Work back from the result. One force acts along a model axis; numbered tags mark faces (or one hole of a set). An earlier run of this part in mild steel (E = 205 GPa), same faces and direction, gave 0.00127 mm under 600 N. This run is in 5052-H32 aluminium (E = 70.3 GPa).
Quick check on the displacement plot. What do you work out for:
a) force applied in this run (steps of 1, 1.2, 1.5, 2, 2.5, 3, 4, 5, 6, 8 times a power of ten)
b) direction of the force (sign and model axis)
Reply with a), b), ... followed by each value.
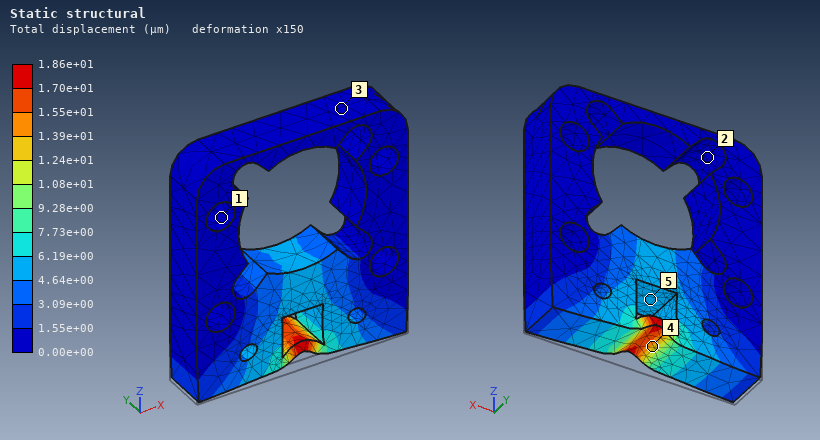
a) 3 kN
b) +Z
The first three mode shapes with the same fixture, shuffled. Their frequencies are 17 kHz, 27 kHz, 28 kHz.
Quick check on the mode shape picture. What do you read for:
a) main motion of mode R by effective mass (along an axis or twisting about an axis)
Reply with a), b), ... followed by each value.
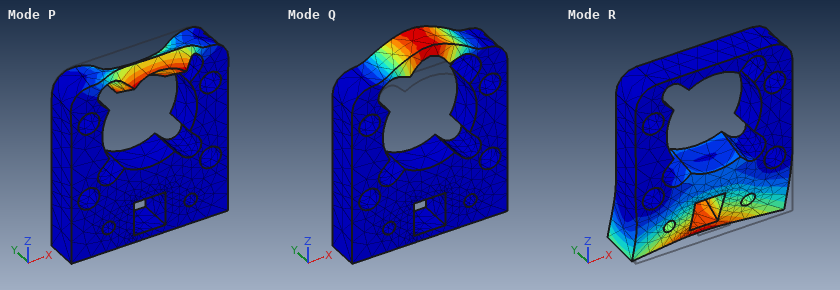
a) along Y
